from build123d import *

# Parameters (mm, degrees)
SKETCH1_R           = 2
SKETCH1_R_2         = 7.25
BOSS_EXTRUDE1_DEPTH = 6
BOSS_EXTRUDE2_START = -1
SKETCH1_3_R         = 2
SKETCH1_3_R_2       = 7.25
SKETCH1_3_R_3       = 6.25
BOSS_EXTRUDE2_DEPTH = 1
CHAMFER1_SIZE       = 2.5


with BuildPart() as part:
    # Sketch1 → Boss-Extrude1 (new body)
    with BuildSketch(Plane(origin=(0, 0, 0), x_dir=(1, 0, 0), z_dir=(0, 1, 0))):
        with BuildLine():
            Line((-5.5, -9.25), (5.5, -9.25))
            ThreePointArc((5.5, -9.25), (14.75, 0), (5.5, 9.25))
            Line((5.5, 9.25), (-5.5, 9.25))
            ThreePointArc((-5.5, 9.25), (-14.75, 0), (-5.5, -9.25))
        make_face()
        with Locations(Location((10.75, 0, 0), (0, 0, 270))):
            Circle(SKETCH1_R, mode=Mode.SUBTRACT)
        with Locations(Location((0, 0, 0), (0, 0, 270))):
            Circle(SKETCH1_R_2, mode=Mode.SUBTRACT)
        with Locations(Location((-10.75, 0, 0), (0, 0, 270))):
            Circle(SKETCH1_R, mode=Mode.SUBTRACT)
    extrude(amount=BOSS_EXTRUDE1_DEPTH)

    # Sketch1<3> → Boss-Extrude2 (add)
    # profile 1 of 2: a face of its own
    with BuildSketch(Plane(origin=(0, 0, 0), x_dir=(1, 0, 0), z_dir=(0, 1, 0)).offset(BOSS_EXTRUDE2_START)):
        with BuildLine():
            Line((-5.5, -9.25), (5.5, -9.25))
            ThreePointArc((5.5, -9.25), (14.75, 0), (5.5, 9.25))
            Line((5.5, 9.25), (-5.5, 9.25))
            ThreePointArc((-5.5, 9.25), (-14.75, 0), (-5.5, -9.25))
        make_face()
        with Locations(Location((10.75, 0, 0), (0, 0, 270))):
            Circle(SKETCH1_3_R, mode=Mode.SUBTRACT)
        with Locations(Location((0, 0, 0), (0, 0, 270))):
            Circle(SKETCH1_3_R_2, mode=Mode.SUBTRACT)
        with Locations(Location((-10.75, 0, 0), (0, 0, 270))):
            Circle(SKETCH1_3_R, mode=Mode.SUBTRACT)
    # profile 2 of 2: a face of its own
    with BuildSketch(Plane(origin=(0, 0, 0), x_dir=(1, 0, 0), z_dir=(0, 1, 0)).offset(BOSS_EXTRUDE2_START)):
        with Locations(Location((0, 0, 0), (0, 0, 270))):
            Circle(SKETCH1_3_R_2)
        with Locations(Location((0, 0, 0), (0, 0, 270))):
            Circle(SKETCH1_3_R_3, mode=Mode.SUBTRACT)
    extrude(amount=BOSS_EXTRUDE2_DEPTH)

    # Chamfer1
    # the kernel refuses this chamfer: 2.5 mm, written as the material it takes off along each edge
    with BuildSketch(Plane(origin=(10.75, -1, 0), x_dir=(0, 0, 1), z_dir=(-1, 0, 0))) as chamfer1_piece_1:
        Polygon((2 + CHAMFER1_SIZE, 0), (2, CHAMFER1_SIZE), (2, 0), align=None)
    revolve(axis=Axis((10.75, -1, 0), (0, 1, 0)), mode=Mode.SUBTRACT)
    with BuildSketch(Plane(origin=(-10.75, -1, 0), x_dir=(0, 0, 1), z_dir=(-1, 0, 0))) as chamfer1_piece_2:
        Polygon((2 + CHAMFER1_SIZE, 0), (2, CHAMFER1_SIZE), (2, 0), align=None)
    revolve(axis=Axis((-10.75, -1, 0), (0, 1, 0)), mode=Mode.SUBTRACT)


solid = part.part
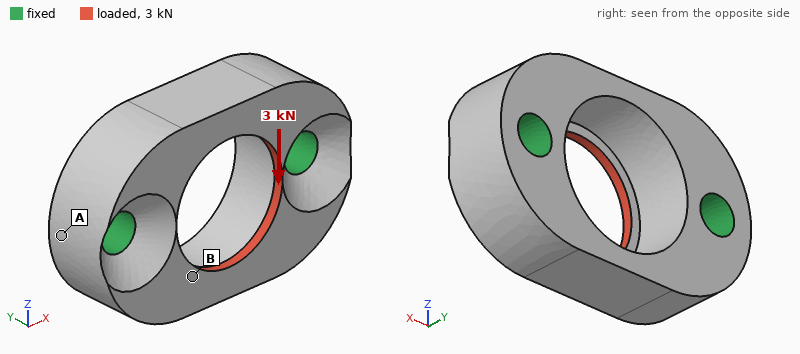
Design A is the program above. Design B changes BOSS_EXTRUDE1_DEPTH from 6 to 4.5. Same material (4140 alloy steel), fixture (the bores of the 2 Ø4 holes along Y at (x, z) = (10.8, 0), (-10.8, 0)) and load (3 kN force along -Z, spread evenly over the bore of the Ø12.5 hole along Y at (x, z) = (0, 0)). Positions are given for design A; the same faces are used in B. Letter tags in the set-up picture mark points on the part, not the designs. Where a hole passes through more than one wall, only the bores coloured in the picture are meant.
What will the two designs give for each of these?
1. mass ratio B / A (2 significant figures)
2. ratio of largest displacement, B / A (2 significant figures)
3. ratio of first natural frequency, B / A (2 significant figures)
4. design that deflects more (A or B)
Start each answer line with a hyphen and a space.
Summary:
- 0.78
- 1.4
- 0.79
- B
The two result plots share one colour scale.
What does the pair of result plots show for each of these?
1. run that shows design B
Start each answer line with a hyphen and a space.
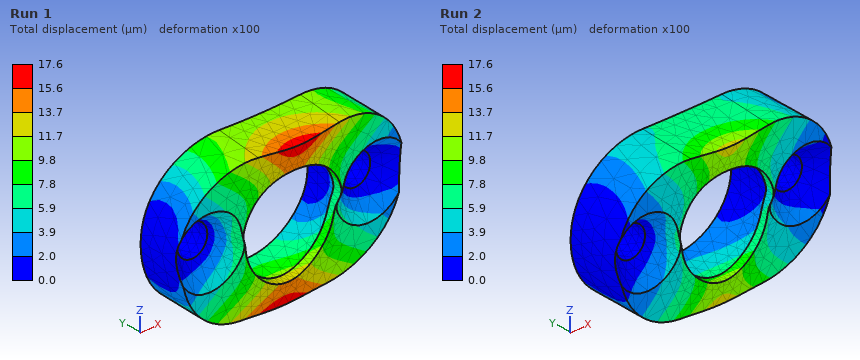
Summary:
- Run 1
